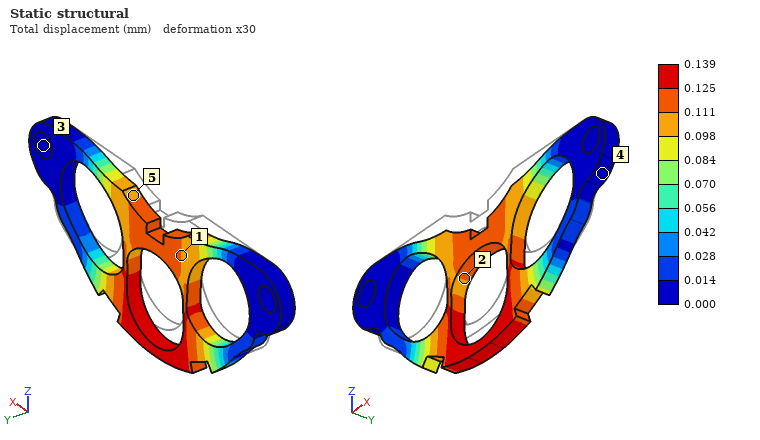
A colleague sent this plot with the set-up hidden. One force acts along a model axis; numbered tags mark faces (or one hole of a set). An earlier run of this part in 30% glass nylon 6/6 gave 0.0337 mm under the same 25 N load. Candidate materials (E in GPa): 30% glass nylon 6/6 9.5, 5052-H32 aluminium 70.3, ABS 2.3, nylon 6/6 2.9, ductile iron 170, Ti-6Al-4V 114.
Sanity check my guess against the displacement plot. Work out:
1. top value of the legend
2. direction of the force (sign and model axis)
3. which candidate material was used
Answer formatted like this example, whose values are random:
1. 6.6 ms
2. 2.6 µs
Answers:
1. 0.139 mm
2. -Z
3. ABS
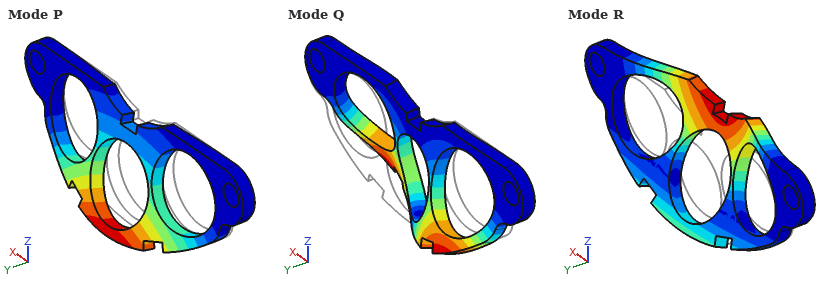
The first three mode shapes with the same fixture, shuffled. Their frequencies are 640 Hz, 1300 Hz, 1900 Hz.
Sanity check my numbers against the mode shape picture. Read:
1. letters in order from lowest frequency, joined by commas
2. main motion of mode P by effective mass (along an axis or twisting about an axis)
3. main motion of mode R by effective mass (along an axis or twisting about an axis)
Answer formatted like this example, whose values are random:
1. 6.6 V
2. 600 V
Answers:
1. P, R, Q
2. along Y
3. along Y
